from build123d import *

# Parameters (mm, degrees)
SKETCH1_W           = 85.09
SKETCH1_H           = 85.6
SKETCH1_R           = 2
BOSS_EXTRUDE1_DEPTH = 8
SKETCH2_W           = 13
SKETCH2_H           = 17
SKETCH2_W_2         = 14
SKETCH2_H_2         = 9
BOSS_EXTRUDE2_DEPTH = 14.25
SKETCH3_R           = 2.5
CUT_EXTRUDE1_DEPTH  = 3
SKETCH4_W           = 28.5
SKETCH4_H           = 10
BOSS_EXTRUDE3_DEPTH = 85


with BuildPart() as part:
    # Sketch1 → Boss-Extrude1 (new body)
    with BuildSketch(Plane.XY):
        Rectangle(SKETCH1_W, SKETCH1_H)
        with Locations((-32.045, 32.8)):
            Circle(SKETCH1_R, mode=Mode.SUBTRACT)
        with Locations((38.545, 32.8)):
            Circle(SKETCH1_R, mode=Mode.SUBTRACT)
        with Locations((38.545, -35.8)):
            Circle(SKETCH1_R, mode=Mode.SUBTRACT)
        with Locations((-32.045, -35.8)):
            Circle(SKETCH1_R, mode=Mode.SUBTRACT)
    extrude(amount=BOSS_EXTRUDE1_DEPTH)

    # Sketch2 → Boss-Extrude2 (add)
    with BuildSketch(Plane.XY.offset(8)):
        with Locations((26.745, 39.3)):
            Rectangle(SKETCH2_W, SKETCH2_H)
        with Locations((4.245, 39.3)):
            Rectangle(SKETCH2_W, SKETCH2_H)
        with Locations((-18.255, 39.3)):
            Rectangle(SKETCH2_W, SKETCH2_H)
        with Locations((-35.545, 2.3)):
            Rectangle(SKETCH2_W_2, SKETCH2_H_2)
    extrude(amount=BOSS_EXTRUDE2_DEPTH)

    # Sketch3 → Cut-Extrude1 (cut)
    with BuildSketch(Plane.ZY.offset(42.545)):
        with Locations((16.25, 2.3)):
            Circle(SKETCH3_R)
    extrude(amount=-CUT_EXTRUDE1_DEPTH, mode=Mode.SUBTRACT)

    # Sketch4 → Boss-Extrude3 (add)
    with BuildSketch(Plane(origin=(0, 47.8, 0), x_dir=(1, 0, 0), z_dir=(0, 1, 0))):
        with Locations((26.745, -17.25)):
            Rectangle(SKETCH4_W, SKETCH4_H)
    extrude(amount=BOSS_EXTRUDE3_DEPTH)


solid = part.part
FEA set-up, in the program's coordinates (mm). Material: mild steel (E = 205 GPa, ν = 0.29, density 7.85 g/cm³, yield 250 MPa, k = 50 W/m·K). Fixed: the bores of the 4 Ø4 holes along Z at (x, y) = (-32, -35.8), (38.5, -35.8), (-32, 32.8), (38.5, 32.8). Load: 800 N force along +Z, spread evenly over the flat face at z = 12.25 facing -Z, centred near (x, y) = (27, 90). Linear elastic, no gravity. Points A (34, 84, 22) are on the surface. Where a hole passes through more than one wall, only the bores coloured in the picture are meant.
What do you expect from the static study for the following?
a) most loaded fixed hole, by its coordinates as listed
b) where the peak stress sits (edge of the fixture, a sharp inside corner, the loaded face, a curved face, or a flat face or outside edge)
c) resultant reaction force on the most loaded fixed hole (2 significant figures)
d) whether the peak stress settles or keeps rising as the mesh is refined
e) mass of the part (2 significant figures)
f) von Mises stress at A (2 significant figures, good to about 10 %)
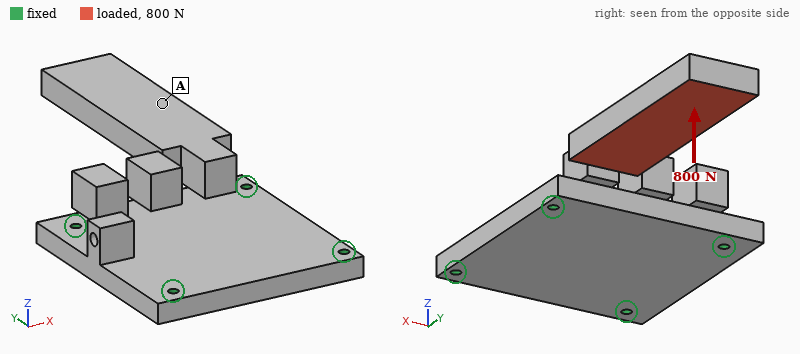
(38.5, 32.8)
edge of the fixture
980 N
keeps rising
730 g
24 MPa
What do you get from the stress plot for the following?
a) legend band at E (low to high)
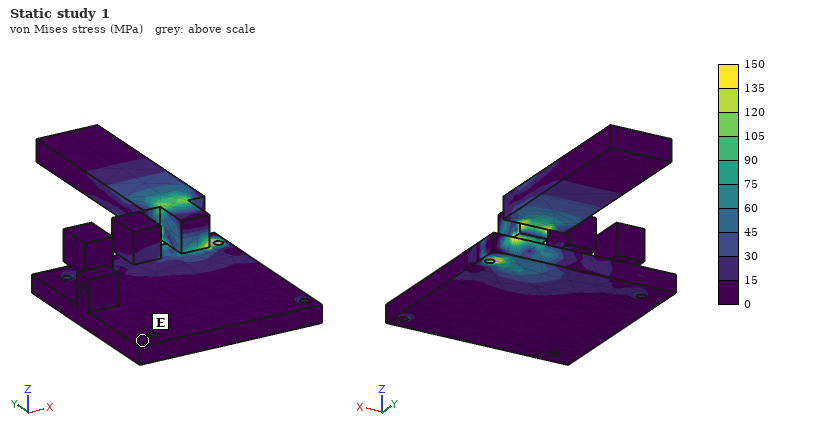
0 to 15 MPa
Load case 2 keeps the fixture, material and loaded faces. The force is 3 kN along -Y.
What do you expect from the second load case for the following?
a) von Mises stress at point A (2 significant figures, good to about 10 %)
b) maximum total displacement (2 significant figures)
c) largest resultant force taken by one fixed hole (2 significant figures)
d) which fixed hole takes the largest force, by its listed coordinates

12 MPa
30 µm
1.8 kN
(38.5, 32.8)
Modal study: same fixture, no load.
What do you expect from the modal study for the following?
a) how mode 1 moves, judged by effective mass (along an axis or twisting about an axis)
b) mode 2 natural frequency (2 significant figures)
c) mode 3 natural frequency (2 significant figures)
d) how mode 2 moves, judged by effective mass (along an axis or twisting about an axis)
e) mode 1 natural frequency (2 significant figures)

along Z
890 Hz
3300 Hz
along X
610 Hz
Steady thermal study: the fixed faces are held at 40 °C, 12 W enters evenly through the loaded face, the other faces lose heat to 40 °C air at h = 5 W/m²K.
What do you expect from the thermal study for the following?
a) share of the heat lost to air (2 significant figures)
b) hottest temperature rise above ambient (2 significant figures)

13 %
65 K
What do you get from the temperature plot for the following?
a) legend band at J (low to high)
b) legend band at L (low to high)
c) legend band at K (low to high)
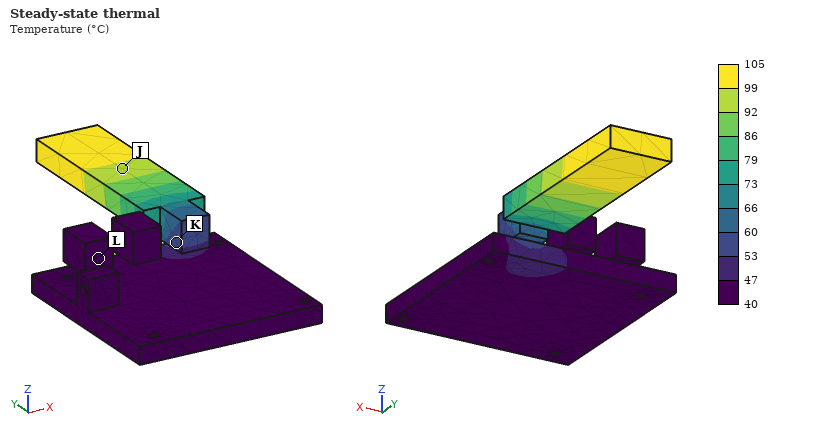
92 to 99 °C
40 to 47 °C
53 to 60 °C
